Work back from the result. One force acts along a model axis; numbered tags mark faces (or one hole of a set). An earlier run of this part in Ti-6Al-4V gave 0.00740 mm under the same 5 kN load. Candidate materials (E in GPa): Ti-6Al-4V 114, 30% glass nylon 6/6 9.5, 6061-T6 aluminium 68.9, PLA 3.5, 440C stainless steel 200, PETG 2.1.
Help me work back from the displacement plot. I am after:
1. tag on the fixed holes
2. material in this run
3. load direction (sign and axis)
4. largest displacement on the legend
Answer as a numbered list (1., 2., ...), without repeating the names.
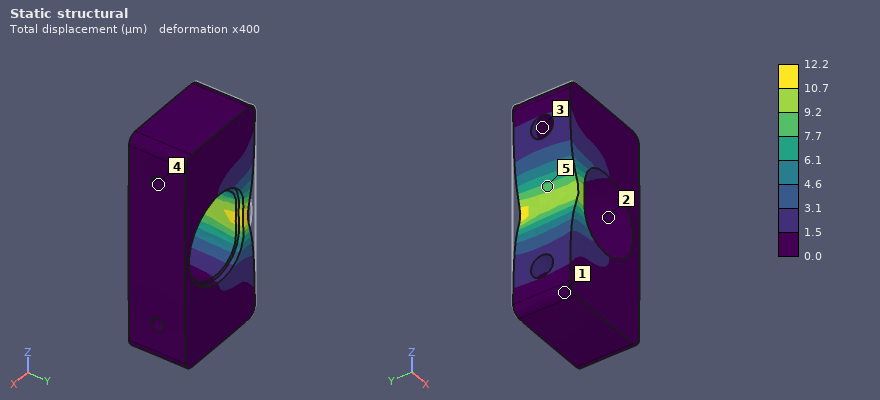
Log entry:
1. 4
2. 6061-T6 aluminium
3. +X
4. 12.2 µm
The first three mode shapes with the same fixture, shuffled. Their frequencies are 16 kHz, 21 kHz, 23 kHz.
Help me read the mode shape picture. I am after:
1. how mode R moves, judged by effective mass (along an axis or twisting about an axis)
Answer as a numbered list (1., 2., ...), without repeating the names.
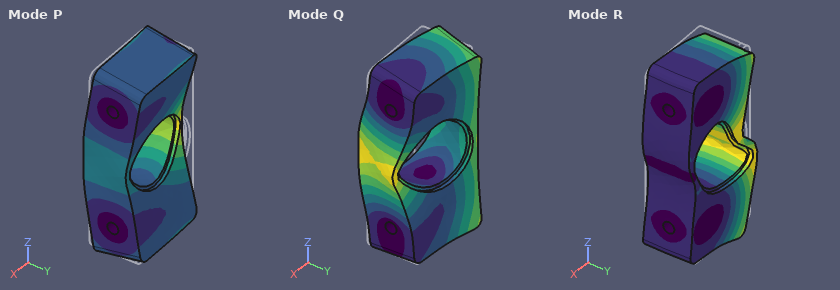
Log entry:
1. along Z
